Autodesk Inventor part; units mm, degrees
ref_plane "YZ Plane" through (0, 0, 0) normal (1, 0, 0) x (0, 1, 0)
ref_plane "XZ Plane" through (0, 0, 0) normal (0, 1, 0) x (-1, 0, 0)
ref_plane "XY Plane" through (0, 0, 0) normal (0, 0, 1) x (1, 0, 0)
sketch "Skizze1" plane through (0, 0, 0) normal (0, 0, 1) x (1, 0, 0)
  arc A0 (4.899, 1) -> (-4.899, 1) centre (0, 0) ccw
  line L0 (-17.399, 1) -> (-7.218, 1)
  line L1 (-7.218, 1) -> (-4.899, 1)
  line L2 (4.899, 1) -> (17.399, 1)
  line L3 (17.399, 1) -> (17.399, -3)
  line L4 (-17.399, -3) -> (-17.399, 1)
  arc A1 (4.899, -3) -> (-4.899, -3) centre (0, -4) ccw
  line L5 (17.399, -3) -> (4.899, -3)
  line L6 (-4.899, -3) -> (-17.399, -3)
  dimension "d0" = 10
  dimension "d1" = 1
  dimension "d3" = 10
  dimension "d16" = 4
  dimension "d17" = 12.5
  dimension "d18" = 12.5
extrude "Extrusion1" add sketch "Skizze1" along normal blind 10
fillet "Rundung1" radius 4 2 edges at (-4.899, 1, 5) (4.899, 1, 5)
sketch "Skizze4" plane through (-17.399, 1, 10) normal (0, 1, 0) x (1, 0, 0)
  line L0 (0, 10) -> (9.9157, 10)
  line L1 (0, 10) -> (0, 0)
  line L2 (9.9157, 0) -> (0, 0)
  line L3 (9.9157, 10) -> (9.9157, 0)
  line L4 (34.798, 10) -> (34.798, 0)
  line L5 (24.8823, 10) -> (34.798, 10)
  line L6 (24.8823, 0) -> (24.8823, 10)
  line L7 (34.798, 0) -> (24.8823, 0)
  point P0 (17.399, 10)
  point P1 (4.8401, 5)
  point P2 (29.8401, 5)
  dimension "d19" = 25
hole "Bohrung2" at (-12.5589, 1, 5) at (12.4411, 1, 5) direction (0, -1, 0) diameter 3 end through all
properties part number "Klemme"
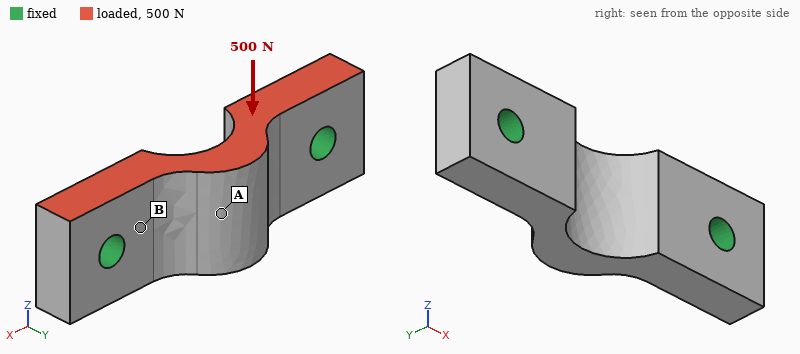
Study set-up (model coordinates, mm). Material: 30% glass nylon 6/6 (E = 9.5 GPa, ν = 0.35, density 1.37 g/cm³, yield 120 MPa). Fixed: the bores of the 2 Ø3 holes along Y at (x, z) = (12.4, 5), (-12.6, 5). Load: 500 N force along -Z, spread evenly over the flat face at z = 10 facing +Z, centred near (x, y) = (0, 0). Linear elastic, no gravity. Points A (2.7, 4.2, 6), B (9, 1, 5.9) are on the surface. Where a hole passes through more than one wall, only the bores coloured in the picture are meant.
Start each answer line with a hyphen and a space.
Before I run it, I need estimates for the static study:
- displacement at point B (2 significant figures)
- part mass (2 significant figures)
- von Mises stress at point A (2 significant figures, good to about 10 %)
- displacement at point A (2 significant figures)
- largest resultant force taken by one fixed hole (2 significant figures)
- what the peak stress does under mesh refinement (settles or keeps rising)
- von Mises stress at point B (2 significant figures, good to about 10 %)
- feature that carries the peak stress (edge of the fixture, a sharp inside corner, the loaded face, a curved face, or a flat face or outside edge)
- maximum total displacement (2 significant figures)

- 10 µm
- 1.9 g
- 5.9 MPa
- 41 µm
- 250 N
- keeps rising
- 17 MPa
- edge of the fixture
- 52 µm
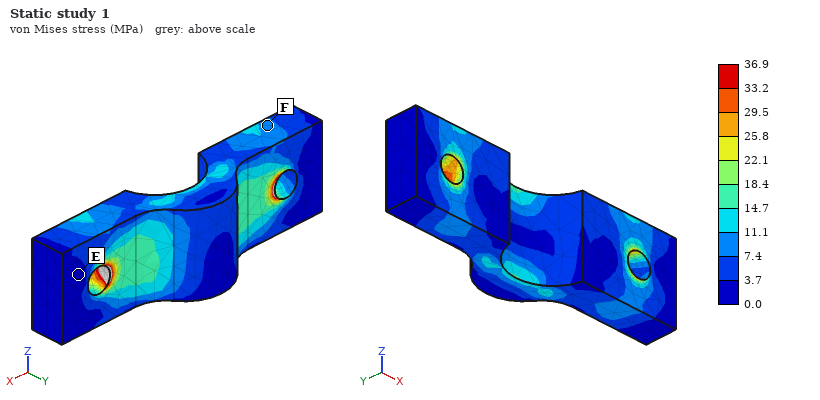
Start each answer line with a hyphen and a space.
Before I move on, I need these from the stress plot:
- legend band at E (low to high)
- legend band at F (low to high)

- 0.0 to 3.7 MPa
- 7.4 to 11.1 MPa
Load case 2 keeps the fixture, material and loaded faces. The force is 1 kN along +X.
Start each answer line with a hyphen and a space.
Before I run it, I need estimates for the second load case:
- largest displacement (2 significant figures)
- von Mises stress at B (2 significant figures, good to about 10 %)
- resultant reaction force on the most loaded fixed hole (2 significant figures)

- 28 µm
- 21 MPa
- 520 N
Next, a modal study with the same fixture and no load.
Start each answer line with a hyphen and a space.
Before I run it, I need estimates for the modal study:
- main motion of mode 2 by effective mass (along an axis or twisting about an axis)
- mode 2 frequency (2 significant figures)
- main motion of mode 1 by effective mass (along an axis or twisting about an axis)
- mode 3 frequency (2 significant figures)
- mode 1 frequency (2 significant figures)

- along Y
- 18 kHz
- along Z
- 27 kHz
- 14 kHz
